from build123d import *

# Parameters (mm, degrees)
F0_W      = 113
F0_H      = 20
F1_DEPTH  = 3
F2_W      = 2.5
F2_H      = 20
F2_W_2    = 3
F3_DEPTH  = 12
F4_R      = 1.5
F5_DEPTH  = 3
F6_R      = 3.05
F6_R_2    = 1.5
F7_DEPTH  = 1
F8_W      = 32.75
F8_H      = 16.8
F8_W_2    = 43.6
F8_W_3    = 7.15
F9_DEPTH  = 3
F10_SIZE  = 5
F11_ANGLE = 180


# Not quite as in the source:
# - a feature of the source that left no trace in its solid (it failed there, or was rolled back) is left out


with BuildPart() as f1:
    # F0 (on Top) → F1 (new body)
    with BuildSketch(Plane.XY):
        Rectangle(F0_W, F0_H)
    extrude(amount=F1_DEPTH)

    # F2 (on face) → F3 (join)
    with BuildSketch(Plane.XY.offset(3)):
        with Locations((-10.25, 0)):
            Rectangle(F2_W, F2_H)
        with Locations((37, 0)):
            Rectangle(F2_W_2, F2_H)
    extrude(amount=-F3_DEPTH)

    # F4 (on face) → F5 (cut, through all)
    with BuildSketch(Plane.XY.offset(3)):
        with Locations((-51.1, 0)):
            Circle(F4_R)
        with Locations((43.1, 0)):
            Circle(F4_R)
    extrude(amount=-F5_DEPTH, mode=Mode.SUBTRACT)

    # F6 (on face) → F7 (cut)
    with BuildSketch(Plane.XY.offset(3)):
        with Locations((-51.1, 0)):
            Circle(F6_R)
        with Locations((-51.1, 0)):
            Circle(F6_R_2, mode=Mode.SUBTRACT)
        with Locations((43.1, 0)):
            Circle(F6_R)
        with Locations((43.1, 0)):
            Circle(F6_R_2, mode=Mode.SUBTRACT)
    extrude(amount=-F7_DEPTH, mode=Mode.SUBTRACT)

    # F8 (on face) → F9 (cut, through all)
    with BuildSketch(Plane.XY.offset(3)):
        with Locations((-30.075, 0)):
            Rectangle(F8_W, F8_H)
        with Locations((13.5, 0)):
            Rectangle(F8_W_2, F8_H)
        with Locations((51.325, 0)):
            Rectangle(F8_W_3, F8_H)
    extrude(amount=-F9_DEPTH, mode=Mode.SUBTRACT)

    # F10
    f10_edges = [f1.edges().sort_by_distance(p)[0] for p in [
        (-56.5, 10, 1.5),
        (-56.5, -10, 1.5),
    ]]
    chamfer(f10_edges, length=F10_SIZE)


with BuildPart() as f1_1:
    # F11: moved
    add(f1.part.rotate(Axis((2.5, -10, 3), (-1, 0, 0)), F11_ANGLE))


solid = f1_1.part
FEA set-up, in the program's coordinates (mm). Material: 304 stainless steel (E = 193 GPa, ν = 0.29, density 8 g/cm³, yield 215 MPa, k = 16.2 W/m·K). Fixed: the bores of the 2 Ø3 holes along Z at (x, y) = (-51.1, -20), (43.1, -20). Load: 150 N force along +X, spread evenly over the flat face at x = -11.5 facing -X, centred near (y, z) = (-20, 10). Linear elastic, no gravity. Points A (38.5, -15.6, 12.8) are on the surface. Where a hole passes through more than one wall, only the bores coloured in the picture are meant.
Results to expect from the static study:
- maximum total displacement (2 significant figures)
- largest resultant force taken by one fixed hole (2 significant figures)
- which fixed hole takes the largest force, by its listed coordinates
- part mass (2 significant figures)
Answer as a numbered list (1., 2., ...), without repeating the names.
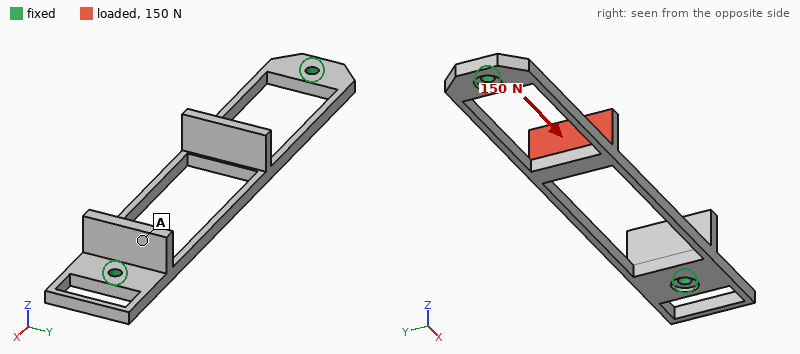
1. 50 µm
2. 83 N
3. (-51.1, -20)
4. 27 g
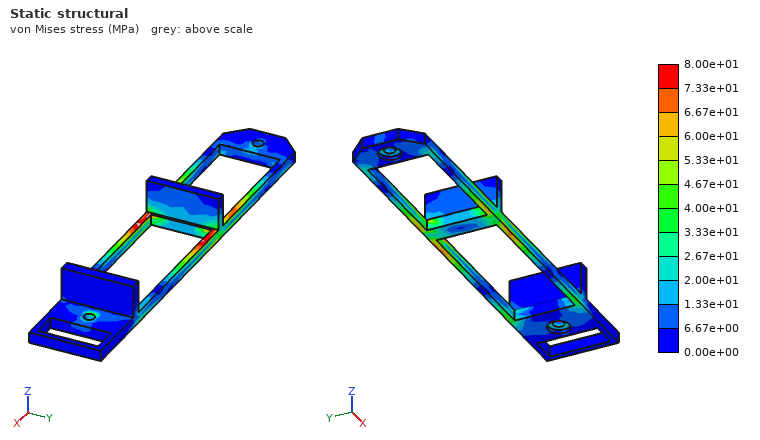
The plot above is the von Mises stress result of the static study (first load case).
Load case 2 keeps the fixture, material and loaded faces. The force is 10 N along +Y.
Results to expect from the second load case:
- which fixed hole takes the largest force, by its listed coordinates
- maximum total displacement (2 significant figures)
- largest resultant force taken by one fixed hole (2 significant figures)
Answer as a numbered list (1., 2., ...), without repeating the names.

1. (-51.1, -20)
2. 70 µm
3. 6.8 N
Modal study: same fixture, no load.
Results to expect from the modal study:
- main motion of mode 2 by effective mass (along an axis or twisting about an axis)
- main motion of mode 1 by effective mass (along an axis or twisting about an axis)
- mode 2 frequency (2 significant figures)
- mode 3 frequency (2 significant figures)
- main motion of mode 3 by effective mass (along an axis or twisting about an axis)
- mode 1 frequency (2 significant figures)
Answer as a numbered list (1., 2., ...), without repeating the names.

1. along Z
2. along Y
3. 1100 Hz
4. 1800 Hz
5. twisting about X
6. 710 Hz
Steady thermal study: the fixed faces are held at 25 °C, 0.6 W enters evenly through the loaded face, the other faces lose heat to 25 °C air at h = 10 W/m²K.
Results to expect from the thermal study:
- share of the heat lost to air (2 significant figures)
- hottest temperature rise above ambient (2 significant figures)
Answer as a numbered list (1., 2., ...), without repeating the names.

1. 71 %
2. 38 K
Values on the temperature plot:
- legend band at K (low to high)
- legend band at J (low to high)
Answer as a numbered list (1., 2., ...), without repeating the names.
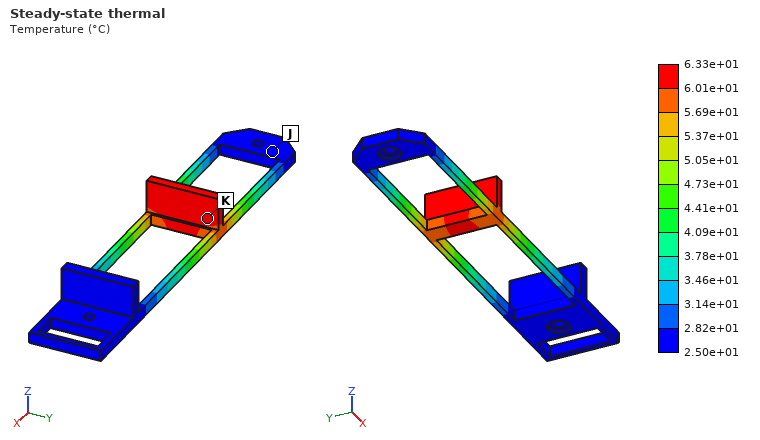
1. 6.01e+01 to 6.33e+01 °C
2. 2.50e+01 to 2.82e+01 °C
